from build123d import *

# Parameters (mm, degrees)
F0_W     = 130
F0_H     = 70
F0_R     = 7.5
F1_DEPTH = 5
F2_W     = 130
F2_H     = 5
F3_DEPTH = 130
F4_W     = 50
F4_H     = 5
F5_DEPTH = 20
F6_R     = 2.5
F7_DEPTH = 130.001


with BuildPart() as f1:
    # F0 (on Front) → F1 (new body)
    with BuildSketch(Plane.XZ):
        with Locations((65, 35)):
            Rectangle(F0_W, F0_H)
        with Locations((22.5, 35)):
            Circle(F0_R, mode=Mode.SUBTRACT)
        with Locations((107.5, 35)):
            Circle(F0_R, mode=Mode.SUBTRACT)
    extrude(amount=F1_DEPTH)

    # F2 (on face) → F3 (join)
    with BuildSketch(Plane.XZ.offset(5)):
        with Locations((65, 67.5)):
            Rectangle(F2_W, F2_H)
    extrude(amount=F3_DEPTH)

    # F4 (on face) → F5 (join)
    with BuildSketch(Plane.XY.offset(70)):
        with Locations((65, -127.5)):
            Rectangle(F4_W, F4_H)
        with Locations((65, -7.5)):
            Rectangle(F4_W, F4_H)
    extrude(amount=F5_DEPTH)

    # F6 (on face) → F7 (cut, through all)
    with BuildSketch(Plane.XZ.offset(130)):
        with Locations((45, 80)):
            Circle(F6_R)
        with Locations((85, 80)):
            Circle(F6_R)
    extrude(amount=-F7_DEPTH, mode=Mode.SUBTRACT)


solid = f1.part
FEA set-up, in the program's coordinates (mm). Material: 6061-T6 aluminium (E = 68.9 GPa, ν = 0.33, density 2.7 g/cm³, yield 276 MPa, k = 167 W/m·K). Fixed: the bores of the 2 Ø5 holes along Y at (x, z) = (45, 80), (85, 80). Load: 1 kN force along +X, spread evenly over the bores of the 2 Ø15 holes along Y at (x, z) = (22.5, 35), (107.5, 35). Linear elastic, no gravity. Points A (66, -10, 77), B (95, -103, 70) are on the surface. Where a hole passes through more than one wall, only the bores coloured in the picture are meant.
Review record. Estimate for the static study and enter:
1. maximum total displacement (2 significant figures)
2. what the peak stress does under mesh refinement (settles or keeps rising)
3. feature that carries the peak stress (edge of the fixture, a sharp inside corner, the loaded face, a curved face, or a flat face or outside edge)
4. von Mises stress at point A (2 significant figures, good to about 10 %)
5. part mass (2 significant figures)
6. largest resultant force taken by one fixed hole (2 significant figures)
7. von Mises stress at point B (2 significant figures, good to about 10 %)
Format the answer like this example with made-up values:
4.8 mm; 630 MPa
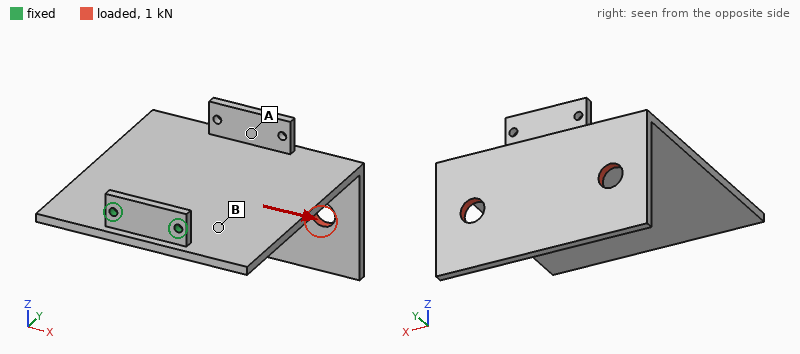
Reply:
2.4 mm; keeps rising; edge of the fixture; 15 MPa; 370 g; 3.3 kN; 40 MPa
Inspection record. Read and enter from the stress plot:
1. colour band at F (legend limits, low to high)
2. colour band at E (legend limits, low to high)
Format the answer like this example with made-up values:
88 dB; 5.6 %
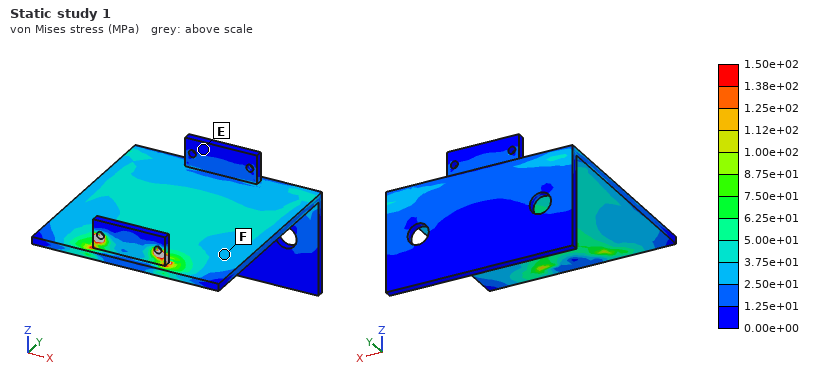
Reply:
2.50e+01 to 3.75e+01 MPa; 0.00e+00 to 1.25e+01 MPa
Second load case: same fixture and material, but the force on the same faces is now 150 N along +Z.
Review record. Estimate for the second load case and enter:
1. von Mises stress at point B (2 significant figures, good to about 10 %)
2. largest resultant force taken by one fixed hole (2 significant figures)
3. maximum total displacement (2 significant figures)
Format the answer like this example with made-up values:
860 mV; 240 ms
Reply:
26 MPa; 160 N; 2.4 mm
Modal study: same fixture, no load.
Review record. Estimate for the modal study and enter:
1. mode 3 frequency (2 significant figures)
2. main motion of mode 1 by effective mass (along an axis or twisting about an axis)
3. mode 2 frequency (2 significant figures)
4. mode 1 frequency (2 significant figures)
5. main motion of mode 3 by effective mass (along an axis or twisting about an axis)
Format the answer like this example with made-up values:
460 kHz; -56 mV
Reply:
470 Hz; along Z; 260 Hz; 97 Hz; along X
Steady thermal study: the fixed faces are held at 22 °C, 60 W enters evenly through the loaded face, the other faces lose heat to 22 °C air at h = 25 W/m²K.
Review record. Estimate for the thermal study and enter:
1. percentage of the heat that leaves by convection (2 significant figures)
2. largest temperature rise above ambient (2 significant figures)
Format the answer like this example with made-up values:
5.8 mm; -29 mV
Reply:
70 %; 56 K
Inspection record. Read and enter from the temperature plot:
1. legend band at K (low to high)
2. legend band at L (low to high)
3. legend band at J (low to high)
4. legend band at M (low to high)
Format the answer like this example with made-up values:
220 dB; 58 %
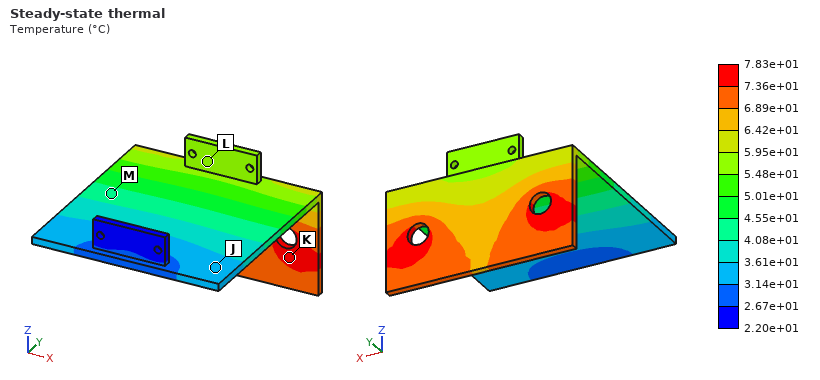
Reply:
7.36e+01 to 7.83e+01 °C; 5.48e+01 to 5.95e+01 °C; 3.14e+01 to 3.61e+01 °C; 4.08e+01 to 4.55e+01 °C
